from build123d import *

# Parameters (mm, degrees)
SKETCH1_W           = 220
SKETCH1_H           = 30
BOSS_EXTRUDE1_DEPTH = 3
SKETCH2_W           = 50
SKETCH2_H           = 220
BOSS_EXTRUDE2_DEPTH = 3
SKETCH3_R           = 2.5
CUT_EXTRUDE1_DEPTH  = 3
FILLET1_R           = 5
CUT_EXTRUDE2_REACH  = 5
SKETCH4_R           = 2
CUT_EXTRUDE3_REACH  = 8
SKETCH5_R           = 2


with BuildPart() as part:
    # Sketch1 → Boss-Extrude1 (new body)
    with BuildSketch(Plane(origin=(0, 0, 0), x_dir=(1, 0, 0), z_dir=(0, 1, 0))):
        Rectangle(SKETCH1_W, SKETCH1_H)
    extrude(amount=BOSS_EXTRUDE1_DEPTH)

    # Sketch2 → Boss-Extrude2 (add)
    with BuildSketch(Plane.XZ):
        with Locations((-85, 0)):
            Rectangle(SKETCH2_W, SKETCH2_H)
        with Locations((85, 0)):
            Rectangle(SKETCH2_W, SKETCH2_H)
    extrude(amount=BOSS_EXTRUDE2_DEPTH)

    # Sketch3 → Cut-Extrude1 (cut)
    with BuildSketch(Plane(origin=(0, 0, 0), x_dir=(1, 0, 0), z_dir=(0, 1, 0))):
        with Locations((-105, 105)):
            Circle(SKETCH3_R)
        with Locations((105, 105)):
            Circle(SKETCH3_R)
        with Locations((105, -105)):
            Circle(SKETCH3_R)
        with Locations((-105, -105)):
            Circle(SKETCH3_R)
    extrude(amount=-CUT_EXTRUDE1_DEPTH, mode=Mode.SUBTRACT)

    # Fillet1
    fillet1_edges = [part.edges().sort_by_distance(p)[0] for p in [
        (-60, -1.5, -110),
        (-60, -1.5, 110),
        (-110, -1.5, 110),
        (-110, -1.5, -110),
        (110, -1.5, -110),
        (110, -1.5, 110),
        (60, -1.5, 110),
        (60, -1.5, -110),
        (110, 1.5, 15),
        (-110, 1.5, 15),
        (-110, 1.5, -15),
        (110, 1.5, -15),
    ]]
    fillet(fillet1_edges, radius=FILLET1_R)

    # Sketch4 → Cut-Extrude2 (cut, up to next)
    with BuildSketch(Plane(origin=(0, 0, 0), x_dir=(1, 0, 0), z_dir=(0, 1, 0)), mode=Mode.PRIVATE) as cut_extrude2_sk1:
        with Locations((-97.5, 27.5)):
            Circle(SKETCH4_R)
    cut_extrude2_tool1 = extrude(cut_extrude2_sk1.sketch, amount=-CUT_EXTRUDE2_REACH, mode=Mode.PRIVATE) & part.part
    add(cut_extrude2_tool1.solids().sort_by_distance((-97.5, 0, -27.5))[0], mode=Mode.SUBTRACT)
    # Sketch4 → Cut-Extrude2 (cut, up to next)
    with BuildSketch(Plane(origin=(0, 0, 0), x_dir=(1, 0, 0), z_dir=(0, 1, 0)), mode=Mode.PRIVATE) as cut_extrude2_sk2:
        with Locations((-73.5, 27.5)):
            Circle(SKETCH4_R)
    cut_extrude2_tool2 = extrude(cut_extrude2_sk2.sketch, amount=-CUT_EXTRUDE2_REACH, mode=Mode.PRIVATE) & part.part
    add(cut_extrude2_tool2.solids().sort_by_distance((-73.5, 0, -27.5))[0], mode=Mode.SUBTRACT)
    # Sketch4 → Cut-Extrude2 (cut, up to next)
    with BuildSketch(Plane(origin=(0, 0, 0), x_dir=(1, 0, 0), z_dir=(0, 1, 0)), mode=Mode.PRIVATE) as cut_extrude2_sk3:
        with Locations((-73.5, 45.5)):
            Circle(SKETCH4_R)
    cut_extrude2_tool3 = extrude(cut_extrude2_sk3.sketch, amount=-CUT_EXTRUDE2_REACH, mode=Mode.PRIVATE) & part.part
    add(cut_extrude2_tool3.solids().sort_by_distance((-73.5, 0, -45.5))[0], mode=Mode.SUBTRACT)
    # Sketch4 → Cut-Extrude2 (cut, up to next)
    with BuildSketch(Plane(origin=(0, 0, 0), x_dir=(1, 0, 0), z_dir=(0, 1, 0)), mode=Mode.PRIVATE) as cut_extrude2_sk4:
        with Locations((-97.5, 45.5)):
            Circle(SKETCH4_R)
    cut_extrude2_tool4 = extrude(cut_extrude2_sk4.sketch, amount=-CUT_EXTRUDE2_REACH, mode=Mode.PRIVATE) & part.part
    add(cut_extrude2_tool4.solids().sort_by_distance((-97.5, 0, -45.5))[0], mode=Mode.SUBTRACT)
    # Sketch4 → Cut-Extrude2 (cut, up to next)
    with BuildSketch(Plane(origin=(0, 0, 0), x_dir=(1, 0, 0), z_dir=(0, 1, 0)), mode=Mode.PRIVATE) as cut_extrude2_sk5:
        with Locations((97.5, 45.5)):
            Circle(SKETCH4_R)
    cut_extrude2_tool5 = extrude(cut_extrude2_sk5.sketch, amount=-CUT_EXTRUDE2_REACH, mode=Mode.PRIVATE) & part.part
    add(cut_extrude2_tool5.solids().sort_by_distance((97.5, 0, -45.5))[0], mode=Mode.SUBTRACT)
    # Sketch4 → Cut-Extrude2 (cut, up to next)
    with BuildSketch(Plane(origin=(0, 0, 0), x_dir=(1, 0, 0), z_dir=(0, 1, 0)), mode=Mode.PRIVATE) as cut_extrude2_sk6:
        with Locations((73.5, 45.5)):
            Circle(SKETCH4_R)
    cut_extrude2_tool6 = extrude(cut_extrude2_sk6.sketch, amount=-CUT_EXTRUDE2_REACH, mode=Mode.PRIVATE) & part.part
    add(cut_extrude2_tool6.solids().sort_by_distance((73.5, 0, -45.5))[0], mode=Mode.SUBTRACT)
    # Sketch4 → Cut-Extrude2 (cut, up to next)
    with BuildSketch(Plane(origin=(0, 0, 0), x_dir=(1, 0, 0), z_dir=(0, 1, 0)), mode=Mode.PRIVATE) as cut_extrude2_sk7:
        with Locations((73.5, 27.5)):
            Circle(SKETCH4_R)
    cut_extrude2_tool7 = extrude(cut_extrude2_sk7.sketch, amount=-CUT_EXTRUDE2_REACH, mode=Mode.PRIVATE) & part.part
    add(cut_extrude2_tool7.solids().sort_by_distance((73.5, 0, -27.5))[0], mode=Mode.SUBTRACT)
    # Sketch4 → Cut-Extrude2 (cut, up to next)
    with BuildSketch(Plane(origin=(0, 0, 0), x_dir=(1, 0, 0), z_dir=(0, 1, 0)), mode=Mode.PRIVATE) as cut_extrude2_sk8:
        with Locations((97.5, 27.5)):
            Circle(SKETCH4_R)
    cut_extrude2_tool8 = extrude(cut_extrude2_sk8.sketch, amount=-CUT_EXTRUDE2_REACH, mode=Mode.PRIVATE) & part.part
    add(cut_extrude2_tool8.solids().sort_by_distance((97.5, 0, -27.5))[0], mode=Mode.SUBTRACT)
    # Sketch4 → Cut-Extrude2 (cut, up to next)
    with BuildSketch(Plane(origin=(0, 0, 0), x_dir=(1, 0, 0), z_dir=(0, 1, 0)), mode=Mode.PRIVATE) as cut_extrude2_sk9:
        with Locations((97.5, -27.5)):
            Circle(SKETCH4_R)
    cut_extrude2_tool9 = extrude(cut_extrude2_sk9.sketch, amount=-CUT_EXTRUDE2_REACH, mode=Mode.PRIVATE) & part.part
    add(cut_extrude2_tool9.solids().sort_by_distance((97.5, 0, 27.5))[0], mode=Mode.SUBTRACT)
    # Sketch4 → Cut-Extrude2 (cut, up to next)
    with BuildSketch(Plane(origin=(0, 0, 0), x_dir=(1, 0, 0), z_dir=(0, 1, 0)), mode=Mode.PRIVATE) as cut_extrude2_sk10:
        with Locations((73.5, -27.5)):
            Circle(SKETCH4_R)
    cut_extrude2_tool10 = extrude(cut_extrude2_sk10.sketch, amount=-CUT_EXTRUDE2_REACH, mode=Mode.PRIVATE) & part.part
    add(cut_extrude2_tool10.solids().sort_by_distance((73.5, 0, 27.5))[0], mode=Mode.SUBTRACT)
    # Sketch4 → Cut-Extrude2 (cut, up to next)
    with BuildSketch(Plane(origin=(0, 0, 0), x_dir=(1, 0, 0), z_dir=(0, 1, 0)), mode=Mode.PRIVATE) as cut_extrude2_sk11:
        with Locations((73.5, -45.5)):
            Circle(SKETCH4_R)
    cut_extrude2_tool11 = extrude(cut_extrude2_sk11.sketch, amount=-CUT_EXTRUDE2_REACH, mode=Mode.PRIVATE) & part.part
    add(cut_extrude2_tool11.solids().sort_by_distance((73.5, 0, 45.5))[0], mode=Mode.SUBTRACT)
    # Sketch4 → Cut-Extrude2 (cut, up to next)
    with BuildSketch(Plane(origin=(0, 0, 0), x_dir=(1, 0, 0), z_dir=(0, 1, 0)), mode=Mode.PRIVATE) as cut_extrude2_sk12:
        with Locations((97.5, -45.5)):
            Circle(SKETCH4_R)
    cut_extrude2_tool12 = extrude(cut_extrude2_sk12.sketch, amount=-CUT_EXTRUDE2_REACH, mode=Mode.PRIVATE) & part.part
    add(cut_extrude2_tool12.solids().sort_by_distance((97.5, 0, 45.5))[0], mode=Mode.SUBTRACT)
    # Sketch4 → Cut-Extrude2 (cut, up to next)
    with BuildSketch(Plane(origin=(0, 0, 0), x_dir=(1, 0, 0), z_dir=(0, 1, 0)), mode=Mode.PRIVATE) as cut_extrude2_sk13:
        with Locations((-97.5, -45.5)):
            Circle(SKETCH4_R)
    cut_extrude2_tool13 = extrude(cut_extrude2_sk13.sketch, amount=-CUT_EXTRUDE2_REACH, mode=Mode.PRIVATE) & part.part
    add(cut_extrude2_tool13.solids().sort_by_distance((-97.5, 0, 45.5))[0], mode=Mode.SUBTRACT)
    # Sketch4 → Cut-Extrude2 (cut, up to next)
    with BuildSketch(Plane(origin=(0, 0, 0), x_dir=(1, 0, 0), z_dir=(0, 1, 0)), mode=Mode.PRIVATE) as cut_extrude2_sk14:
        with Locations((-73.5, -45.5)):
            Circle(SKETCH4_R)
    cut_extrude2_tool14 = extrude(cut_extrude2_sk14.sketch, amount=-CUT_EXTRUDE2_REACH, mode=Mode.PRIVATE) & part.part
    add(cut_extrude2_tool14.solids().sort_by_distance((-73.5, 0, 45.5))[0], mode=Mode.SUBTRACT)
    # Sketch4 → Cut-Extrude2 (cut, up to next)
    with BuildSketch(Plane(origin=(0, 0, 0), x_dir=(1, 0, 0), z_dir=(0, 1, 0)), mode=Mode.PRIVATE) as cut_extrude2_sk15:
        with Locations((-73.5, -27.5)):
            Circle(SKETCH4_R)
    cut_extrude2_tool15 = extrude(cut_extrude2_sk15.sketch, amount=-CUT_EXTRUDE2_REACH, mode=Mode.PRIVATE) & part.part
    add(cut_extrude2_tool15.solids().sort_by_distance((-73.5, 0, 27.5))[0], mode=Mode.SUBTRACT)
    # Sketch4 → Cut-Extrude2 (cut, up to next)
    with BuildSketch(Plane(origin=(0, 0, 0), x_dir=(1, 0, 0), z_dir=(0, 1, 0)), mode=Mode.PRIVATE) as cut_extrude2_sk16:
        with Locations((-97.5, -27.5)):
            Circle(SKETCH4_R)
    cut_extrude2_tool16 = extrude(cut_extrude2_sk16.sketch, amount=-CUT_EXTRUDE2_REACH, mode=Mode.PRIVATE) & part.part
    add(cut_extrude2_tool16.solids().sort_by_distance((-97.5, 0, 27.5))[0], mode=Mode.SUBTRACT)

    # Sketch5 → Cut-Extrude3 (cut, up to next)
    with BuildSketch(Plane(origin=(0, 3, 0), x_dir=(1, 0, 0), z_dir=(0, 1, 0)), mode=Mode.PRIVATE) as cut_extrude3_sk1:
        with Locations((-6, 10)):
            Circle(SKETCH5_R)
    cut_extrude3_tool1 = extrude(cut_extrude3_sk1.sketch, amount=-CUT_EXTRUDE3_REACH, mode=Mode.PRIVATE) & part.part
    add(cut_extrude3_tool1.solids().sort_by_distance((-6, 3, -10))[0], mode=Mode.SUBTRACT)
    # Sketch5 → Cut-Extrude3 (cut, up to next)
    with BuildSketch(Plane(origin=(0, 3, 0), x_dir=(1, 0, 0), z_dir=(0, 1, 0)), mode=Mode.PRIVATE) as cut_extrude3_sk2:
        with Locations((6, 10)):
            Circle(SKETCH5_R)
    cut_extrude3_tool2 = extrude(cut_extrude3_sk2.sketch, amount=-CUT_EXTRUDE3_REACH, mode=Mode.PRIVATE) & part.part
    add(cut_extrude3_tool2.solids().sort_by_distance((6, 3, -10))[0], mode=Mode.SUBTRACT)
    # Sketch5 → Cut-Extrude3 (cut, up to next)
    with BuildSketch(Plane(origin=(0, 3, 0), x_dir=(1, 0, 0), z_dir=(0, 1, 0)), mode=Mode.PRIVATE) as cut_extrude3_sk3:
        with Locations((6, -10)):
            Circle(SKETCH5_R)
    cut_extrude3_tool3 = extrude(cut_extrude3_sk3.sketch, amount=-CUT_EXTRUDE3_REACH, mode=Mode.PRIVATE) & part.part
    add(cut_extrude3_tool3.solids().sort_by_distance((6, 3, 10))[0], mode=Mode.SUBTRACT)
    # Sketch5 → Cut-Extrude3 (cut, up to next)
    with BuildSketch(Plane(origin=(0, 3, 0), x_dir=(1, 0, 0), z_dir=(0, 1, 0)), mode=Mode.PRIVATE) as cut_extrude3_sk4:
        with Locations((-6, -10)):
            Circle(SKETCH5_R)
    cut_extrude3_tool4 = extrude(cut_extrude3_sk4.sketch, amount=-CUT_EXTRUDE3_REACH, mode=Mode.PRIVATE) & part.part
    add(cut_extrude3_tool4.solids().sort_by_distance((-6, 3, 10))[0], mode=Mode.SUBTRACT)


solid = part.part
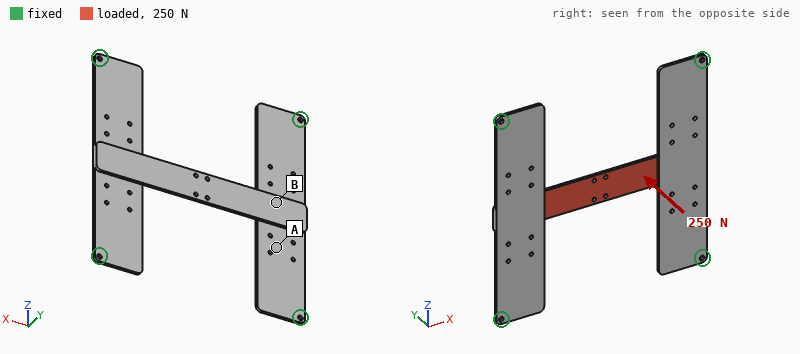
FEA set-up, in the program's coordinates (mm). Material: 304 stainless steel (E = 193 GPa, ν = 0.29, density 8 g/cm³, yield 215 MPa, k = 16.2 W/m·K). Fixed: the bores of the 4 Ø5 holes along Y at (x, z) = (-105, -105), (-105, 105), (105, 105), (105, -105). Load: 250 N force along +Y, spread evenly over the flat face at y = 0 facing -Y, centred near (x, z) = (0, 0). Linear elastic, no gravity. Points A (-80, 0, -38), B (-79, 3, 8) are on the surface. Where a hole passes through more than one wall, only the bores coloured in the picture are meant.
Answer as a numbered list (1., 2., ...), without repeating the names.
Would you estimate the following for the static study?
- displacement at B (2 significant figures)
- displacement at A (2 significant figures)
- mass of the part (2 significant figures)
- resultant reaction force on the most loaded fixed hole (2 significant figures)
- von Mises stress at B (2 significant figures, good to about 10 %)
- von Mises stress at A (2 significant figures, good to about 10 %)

1. 0.36 mm
2. 0.30 mm
3. 680 g
4. 730 N
5. 13 MPa
6. 30 MPa
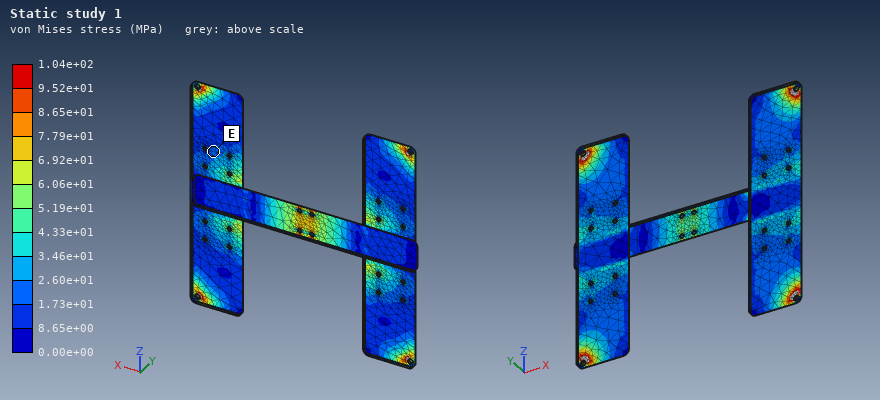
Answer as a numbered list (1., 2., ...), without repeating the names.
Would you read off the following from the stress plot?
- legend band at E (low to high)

1. 1.73e+01 to 2.60e+01 MPa
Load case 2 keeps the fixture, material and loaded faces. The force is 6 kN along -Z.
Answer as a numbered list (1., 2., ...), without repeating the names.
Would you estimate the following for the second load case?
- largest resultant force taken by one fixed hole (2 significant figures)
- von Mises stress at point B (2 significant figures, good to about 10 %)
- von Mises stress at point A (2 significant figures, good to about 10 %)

1. 1.7 kN
2. 21 MPa
3. 32 MPa
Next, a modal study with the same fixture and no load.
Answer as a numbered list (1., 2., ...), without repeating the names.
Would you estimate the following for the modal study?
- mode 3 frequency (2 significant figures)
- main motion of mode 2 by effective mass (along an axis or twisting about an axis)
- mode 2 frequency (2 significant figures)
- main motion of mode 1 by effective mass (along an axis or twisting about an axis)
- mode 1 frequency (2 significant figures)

1. 550 Hz
2. twisting about Z
3. 290 Hz
4. along Y
5. 220 Hz
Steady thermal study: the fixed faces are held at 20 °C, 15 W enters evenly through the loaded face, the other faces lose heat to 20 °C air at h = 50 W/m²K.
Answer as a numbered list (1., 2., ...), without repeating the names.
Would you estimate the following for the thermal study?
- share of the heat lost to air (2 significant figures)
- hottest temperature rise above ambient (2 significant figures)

1. 100 %
2. 56 K
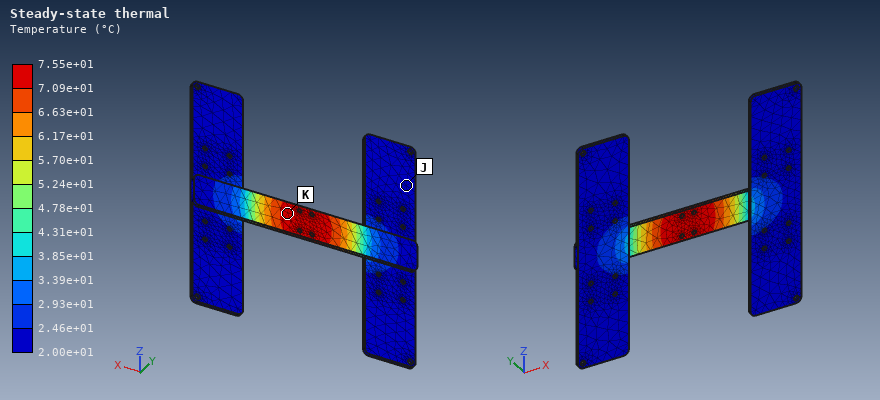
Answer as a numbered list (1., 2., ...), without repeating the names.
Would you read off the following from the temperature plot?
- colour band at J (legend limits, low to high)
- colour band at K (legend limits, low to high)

1. 2.00e+01 to 2.46e+01 °C
2. 7.09e+01 to 7.55e+01 °C
